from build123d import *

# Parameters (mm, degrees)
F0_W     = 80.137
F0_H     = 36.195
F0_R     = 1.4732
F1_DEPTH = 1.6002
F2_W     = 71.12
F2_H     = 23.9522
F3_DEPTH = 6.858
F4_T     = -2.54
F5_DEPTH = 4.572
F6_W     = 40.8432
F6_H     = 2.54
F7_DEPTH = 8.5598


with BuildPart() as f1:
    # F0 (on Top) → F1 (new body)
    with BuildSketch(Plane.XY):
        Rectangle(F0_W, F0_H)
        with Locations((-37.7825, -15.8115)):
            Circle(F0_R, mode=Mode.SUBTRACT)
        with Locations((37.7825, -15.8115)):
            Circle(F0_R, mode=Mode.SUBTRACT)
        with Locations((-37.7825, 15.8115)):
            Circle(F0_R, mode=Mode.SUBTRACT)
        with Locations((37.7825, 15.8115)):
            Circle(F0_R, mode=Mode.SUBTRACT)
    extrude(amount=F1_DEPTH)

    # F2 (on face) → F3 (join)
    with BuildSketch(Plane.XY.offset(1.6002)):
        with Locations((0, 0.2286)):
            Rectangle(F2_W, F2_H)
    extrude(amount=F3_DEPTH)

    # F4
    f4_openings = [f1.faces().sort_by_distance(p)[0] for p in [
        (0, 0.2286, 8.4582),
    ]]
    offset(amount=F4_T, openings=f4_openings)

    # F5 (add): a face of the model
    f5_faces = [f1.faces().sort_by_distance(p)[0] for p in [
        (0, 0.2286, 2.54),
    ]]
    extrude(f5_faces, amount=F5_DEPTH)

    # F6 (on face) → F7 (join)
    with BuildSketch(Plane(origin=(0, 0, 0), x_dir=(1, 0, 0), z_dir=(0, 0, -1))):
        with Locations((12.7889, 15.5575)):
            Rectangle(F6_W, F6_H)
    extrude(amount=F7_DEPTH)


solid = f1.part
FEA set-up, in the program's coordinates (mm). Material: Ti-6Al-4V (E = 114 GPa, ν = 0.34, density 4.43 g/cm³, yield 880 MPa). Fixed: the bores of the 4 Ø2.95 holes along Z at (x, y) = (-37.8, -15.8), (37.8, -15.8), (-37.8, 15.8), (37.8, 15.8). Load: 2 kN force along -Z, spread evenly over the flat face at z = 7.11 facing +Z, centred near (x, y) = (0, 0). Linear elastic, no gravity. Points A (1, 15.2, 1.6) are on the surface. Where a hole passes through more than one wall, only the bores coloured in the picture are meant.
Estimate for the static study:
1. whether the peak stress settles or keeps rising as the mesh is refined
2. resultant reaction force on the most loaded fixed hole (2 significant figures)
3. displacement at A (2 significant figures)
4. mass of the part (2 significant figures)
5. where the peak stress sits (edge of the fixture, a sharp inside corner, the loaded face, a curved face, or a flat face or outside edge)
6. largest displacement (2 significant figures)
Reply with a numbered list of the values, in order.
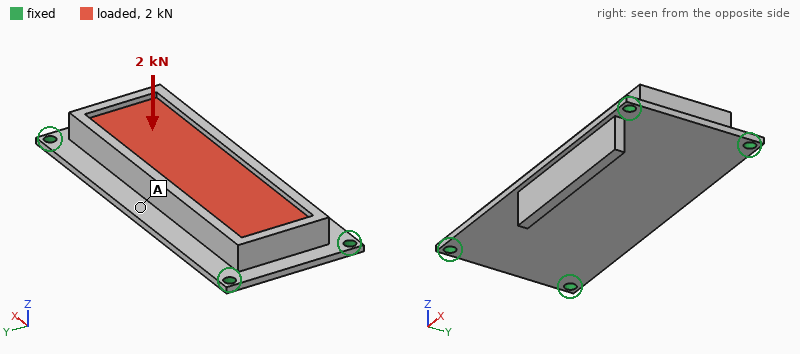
1. keeps rising
2. 1.0 kN
3. 90 µm
4. 69 g
5. edge of the fixture
6. 93 µm
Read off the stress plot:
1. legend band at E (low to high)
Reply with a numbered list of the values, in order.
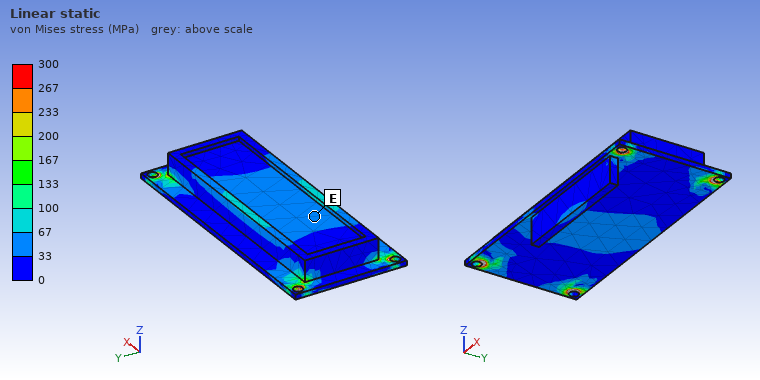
1. 33 to 67 MPa
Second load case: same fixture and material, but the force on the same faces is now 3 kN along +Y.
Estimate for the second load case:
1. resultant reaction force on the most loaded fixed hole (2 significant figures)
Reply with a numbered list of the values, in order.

1. 1.1 kN
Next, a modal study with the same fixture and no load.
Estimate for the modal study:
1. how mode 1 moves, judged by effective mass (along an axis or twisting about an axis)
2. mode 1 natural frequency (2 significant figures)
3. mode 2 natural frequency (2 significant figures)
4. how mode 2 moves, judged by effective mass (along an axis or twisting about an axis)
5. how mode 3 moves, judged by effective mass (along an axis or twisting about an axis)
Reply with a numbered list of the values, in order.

1. along Z
2. 3400 Hz
3. 6100 Hz
4. twisting about X
5. twisting about Y
